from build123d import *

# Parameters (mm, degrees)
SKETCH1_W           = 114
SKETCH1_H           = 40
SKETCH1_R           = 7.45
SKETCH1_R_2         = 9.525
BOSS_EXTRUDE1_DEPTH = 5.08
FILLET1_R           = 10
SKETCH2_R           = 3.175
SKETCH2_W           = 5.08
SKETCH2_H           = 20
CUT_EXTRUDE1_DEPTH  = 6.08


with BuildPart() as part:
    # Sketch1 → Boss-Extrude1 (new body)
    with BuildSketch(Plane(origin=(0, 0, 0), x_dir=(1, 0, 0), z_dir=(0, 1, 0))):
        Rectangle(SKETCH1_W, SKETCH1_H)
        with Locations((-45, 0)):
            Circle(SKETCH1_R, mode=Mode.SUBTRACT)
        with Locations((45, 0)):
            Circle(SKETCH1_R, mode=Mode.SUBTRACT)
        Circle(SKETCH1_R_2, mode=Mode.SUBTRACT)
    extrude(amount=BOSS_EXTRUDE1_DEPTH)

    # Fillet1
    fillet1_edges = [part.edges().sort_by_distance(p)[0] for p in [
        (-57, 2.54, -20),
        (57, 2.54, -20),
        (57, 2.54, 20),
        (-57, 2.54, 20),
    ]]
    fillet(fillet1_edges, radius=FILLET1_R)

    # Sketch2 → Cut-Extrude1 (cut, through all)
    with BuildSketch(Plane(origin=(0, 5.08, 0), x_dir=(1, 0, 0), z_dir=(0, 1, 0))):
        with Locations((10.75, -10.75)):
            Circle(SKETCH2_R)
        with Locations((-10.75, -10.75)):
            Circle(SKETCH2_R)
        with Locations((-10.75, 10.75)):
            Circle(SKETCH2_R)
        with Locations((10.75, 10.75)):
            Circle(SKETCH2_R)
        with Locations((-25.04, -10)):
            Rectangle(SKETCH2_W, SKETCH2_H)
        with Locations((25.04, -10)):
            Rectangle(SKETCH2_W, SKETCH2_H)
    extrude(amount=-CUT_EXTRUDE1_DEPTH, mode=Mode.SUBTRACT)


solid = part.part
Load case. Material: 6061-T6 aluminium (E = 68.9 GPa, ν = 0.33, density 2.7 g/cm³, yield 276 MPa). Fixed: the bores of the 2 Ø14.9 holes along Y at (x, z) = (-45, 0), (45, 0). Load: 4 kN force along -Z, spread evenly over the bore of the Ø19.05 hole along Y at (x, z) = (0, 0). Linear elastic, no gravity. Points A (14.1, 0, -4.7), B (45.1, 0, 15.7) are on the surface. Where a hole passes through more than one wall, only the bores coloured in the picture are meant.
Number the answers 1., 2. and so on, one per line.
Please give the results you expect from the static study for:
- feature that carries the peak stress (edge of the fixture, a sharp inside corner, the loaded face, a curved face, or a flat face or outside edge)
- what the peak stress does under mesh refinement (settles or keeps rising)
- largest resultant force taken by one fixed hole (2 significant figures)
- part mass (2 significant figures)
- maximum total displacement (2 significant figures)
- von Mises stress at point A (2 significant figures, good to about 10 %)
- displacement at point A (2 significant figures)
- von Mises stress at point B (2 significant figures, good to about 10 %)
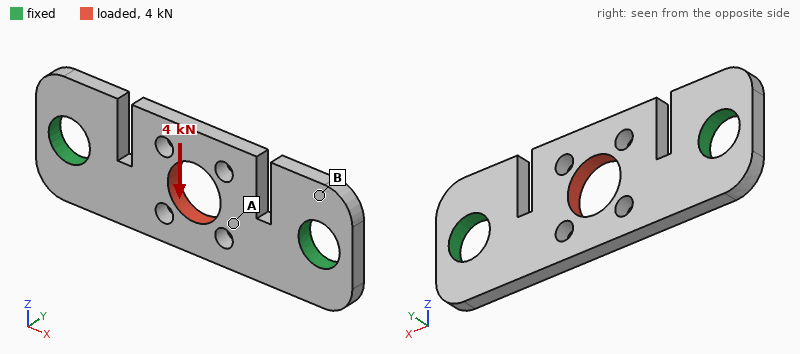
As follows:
1. a sharp inside corner
2. keeps rising
3. 2.1 kN
4. 48 g
5. 47 µm
6. 21 MPa
7. 35 µm
8. 6.5 MPa
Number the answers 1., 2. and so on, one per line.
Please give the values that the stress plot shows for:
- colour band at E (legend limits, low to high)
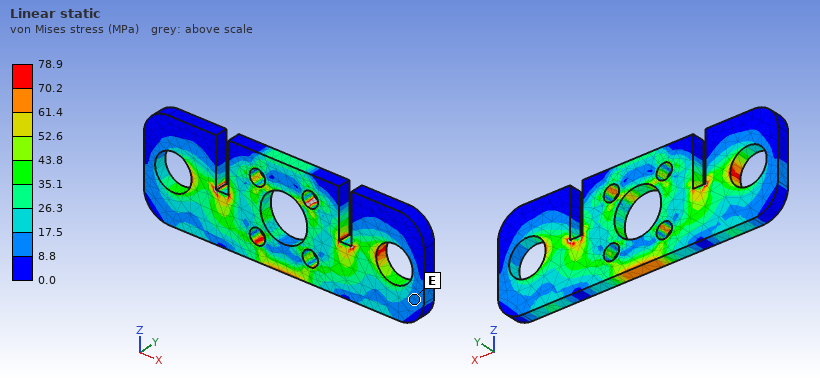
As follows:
1. 8.8 to 17.5 MPa
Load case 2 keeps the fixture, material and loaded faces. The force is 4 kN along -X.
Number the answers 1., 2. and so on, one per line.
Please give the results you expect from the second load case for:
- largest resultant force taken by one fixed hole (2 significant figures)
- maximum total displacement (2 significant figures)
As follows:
1. 2.0 kN
2. 29 µm
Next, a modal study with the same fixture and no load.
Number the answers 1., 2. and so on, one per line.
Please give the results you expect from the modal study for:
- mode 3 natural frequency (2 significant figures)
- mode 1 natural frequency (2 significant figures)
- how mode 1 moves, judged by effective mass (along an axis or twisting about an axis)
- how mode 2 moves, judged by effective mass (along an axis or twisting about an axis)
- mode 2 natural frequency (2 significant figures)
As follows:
1. 6700 Hz
2. 2800 Hz
3. along Y
4. along Y
5. 4400 Hz
